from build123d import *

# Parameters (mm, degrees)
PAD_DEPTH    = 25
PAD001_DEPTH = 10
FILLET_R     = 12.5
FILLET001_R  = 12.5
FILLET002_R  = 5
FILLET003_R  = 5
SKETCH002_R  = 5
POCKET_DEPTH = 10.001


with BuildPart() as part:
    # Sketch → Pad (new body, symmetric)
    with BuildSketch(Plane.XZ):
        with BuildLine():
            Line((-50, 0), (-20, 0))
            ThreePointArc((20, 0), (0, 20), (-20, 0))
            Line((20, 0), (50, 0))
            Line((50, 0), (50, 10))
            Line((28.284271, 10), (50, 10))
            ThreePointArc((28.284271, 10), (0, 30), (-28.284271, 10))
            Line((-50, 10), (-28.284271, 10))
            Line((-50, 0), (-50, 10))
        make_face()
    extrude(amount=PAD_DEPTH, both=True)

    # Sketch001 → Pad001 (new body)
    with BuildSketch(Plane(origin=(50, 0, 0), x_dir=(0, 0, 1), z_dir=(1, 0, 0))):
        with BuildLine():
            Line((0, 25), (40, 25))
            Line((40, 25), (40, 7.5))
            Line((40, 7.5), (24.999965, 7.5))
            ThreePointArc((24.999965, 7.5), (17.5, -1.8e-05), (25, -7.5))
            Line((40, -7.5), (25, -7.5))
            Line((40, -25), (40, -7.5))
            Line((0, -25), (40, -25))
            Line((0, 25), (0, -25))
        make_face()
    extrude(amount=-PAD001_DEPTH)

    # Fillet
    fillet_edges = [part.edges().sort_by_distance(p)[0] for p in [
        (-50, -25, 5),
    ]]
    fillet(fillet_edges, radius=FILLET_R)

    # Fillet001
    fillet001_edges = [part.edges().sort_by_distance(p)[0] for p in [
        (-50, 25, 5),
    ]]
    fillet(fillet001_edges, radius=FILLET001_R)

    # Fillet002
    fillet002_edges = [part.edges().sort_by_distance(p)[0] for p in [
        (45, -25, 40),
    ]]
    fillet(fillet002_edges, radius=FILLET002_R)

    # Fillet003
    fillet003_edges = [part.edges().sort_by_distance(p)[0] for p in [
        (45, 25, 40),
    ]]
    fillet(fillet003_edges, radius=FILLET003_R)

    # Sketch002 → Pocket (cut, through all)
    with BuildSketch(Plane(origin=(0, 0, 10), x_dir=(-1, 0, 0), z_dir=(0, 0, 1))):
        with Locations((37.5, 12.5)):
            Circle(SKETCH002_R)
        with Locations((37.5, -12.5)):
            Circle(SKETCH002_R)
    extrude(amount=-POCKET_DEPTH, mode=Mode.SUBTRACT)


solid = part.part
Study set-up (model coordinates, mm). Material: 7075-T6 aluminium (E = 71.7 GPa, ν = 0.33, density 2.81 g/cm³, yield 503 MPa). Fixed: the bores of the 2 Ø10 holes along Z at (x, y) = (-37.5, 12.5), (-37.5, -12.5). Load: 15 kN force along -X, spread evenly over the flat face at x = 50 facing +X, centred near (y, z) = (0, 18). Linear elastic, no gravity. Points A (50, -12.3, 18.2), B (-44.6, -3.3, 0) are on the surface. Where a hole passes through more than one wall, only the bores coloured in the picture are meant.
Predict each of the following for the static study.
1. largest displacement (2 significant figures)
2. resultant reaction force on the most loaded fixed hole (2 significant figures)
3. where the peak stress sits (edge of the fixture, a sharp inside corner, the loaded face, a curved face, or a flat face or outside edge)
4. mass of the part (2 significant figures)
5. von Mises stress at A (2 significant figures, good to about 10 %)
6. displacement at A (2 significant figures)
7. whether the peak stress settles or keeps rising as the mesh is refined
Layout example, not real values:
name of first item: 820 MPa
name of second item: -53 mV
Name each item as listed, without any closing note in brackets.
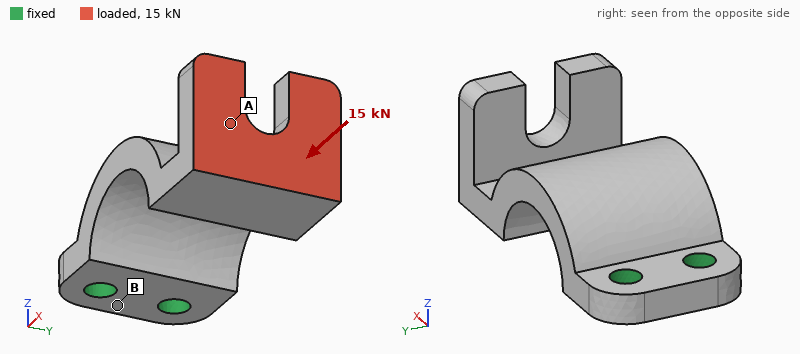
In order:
largest displacement: 1.1 mm
resultant reaction force on the most loaded fixed hole: 7.6 kN
where the peak stress sits: edge of the fixture
mass of the part: 190 g
von Mises stress at A: 110 MPa
displacement at A: 0.76 mm
whether the peak stress settles or keeps rising as the mesh is refined: keeps rising
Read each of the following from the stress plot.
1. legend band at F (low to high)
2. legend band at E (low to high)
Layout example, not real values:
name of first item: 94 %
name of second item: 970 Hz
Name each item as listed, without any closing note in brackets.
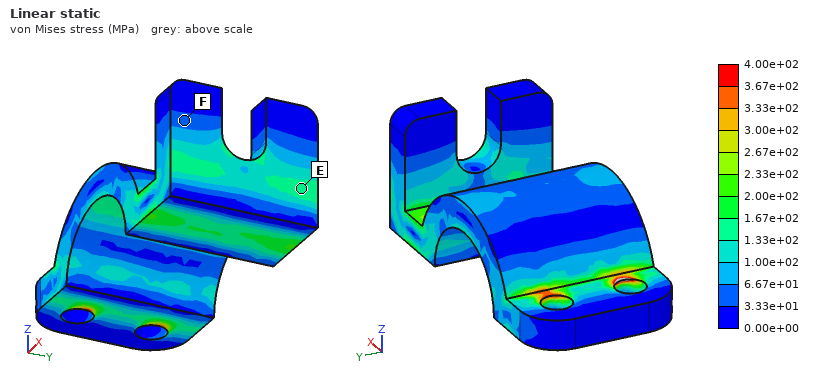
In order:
legend band at F: 3.33e+01 to 6.67e+01 MPa
legend band at E: 1.33e+02 to 1.67e+02 MPa
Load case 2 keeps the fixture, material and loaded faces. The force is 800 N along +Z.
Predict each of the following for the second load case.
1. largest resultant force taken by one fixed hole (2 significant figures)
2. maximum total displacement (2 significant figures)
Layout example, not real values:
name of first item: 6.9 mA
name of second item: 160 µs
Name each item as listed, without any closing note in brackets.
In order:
largest resultant force taken by one fixed hole: 400 N
maximum total displacement: 0.70 mm
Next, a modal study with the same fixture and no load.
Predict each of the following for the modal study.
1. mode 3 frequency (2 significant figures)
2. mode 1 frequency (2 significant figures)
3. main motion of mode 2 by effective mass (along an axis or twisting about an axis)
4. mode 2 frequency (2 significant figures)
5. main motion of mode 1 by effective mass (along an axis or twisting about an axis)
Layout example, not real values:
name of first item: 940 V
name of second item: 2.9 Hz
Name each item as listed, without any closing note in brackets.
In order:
mode 3 frequency: 2600 Hz
mode 1 frequency: 700 Hz
main motion of mode 2 by effective mass: along Y
mode 2 frequency: 1500 Hz
main motion of mode 1 by effective mass: along Z
